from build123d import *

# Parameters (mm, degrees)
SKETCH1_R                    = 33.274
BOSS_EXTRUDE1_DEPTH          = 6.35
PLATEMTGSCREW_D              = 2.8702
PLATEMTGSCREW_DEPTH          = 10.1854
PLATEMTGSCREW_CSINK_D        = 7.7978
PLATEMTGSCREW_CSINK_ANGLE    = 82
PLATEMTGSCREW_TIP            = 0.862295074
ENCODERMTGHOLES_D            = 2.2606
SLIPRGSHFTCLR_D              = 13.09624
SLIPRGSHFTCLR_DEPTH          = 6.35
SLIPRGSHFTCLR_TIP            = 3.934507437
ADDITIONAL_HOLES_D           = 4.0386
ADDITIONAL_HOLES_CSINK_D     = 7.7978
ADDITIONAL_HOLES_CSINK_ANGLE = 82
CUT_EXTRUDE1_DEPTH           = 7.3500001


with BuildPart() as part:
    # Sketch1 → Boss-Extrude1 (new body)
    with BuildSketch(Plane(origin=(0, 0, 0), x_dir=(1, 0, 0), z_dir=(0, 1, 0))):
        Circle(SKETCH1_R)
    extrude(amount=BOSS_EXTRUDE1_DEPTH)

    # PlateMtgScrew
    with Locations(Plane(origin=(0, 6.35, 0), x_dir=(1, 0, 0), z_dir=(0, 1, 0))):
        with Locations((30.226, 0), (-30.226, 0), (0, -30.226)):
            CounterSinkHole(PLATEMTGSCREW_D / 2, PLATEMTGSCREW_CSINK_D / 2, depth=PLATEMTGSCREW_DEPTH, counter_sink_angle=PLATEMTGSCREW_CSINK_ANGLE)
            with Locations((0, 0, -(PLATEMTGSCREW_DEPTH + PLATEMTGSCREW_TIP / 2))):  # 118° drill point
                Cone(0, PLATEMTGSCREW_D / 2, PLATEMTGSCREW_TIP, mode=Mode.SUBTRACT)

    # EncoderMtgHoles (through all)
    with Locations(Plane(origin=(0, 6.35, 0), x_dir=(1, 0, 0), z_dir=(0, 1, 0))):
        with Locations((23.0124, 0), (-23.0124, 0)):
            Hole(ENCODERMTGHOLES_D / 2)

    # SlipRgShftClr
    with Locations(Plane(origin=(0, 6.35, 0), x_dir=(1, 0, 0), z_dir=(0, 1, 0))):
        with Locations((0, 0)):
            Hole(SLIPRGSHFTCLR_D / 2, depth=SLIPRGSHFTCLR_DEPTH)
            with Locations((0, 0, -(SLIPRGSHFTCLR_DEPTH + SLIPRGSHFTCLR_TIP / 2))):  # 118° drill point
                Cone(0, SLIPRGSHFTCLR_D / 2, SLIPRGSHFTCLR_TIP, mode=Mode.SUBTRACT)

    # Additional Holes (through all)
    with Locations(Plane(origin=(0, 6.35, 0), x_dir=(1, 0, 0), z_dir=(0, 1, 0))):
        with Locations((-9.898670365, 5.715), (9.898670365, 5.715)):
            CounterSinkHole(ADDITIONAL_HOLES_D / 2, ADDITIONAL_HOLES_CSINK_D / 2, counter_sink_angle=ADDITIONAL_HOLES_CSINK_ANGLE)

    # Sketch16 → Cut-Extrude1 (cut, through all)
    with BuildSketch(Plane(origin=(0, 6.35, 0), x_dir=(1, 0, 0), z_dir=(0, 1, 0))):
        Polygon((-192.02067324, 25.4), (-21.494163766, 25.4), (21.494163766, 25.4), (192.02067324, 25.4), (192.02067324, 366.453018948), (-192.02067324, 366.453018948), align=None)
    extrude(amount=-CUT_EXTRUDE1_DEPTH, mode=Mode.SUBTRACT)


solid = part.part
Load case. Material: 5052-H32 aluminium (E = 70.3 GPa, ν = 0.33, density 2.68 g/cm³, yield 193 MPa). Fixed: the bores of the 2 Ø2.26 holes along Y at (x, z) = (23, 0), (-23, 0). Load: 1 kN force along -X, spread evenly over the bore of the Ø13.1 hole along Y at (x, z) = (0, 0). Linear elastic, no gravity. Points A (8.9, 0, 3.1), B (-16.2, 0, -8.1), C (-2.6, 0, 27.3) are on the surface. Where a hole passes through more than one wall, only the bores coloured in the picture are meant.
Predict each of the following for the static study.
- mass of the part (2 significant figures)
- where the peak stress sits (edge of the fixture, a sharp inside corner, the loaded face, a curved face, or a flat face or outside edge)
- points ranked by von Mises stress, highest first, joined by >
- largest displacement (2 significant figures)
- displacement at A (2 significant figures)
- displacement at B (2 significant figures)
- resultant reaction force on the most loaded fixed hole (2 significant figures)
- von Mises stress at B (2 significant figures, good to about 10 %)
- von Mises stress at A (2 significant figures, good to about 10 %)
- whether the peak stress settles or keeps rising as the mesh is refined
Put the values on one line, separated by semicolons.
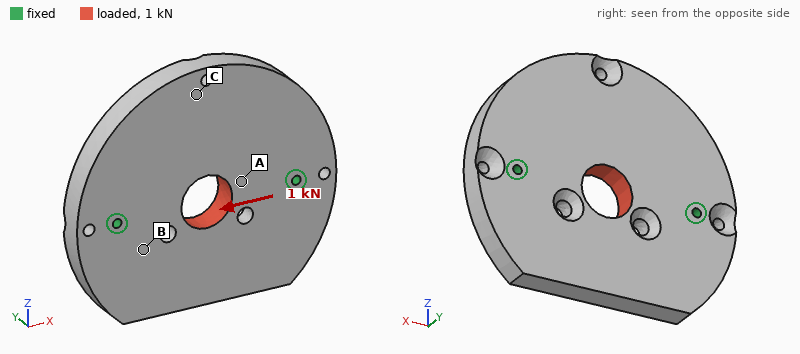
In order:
51 g; edge of the fixture; A > B > C; 2.1 µm; 1.2 µm; 0.98 µm; 500 N; 2.9 MPa; 4.3 MPa; keeps rising
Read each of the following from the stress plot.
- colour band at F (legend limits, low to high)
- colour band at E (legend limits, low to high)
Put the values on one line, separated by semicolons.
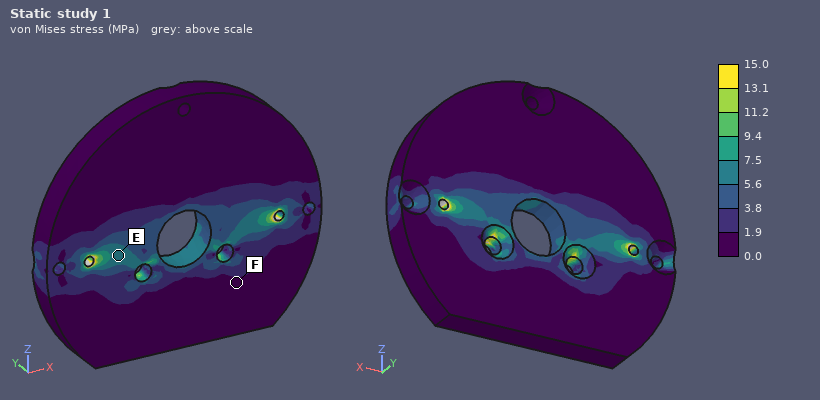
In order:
0.0 to 1.9 MPa; 5.6 to 7.5 MPa
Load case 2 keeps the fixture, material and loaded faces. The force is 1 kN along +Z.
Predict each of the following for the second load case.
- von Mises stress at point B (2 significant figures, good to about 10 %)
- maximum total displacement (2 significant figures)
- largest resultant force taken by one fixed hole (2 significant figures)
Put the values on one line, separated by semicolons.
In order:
3.9 MPa; 2.4 µm; 500 N
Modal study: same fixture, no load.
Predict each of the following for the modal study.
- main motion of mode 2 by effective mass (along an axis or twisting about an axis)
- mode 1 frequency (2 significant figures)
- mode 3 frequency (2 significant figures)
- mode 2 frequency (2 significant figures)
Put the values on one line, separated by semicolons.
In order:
along Y; 3800 Hz; 9600 Hz; 5800 Hz
